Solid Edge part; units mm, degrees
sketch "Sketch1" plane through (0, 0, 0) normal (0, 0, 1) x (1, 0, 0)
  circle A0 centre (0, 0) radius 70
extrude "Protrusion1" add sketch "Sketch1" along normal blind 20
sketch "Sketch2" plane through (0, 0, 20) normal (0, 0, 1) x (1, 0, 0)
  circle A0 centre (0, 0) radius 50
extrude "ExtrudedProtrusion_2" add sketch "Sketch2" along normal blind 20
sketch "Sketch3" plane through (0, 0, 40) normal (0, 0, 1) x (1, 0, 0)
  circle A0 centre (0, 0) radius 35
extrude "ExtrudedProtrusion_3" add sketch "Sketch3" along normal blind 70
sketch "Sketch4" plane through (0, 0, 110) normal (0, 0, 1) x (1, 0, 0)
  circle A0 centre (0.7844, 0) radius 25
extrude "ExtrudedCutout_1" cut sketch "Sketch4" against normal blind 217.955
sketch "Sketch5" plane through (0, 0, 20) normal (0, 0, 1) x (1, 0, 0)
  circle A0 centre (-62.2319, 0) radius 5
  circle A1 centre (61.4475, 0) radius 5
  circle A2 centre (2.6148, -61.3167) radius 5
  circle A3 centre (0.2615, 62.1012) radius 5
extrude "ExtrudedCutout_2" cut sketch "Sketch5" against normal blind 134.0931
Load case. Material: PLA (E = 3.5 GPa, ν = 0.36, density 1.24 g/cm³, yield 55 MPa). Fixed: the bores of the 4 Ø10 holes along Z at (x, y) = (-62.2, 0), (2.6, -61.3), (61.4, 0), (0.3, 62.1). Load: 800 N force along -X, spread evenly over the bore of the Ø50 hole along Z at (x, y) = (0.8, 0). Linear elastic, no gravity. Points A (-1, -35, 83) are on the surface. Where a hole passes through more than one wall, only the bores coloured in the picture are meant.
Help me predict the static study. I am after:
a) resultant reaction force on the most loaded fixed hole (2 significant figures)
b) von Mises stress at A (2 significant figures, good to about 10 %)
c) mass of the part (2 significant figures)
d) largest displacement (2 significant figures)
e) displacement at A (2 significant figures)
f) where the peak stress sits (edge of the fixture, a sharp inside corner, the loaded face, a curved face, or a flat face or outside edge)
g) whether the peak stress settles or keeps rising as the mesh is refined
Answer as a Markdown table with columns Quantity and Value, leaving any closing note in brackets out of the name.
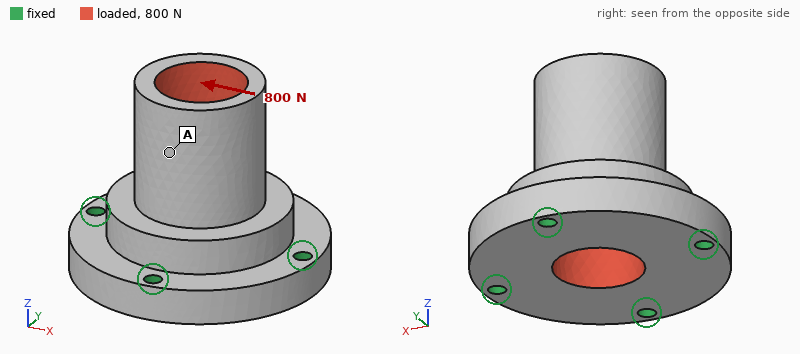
| Quantity | Value |
|---|---|
| resultant reaction force on the most loaded fixed hole | 410 N |
| von Mises stress at A | 0.33 MPa |
| mass of the part | 630 g |
| largest displacement | 47 µm |
| displacement at A | 32 µm |
| where the peak stress sits | edge of the fixture |
| whether the peak stress settles or keeps rising as the mesh is refined | keeps rising |
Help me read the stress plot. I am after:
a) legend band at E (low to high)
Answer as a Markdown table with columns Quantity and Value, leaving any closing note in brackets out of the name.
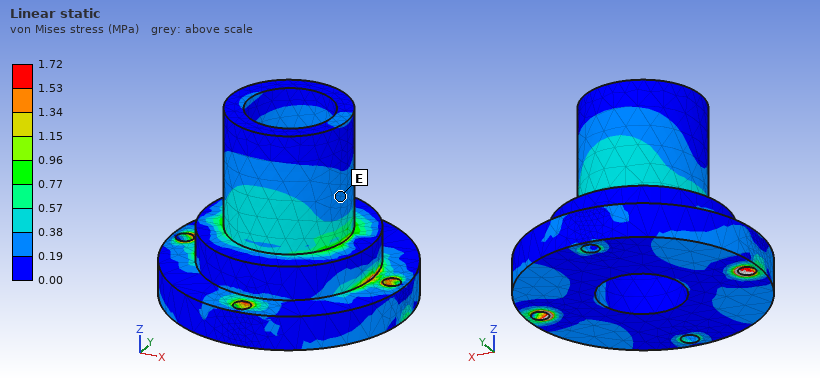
| Quantity | Value |
|---|---|
| legend band at E | 0.19 to 0.38 MPa |
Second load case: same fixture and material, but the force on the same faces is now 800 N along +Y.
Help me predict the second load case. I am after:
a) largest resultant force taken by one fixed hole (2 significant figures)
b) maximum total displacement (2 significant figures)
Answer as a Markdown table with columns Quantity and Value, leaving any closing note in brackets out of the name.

| Quantity | Value |
|---|---|
| largest resultant force taken by one fixed hole | 410 N |
| maximum total displacement | 47 µm |
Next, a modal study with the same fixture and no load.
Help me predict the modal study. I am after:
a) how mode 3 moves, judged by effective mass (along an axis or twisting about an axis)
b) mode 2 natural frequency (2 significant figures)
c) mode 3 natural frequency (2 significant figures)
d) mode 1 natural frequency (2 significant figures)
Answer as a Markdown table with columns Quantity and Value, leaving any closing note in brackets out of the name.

| Quantity | Value |
|---|---|
| how mode 3 moves, judged by effective mass | along Z |
| mode 2 natural frequency | 1500 Hz |
| mode 3 natural frequency | 2300 Hz |
| mode 1 natural frequency | 1500 Hz |
